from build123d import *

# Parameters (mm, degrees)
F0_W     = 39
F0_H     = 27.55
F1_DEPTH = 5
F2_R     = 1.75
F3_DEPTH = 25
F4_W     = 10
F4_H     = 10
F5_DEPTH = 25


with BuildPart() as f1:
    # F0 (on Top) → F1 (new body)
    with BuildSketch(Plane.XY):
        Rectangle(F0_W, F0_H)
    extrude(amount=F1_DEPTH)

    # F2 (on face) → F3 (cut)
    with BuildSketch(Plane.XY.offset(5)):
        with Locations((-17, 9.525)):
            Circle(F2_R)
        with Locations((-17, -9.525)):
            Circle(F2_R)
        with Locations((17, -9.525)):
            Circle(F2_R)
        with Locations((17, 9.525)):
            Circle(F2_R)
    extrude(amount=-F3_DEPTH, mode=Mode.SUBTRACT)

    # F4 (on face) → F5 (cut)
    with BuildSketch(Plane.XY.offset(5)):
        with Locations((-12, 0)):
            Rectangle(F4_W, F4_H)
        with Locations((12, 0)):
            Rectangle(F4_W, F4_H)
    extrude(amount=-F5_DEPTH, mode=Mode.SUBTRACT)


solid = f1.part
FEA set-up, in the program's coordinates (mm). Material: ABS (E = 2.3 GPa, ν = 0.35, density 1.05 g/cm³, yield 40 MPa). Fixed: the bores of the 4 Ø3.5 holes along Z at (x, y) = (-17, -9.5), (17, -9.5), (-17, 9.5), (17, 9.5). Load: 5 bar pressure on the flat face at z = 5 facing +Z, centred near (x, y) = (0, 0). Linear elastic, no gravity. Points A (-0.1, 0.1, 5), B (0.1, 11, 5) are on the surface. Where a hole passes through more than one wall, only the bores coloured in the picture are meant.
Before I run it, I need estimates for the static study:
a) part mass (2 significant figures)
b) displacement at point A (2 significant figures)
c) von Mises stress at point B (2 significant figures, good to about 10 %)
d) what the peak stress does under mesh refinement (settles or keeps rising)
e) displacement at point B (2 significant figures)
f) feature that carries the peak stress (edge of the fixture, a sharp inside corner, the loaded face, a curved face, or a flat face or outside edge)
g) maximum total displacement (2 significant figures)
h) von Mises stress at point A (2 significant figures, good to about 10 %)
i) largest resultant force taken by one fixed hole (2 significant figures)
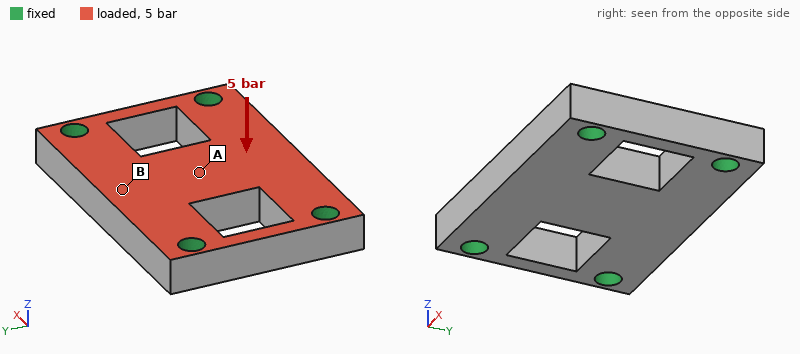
4.4 g
0.10 mm
6.1 MPa
keeps rising
0.094 mm
edge of the fixture
0.10 mm
3.2 MPa
100 N
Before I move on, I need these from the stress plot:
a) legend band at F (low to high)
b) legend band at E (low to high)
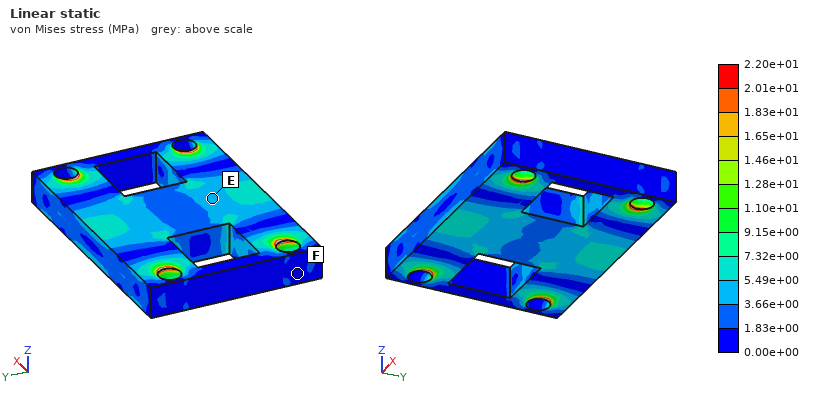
0.00e+00 to 1.83e+00 MPa
3.66e+00 to 5.49e+00 MPa
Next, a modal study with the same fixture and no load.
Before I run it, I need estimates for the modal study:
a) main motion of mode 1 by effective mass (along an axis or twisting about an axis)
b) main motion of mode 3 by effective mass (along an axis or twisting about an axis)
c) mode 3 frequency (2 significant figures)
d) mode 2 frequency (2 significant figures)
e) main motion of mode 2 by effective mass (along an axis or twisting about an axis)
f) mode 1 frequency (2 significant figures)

along Z
along Y
7400 Hz
7000 Hz
twisting about X
5400 Hz
